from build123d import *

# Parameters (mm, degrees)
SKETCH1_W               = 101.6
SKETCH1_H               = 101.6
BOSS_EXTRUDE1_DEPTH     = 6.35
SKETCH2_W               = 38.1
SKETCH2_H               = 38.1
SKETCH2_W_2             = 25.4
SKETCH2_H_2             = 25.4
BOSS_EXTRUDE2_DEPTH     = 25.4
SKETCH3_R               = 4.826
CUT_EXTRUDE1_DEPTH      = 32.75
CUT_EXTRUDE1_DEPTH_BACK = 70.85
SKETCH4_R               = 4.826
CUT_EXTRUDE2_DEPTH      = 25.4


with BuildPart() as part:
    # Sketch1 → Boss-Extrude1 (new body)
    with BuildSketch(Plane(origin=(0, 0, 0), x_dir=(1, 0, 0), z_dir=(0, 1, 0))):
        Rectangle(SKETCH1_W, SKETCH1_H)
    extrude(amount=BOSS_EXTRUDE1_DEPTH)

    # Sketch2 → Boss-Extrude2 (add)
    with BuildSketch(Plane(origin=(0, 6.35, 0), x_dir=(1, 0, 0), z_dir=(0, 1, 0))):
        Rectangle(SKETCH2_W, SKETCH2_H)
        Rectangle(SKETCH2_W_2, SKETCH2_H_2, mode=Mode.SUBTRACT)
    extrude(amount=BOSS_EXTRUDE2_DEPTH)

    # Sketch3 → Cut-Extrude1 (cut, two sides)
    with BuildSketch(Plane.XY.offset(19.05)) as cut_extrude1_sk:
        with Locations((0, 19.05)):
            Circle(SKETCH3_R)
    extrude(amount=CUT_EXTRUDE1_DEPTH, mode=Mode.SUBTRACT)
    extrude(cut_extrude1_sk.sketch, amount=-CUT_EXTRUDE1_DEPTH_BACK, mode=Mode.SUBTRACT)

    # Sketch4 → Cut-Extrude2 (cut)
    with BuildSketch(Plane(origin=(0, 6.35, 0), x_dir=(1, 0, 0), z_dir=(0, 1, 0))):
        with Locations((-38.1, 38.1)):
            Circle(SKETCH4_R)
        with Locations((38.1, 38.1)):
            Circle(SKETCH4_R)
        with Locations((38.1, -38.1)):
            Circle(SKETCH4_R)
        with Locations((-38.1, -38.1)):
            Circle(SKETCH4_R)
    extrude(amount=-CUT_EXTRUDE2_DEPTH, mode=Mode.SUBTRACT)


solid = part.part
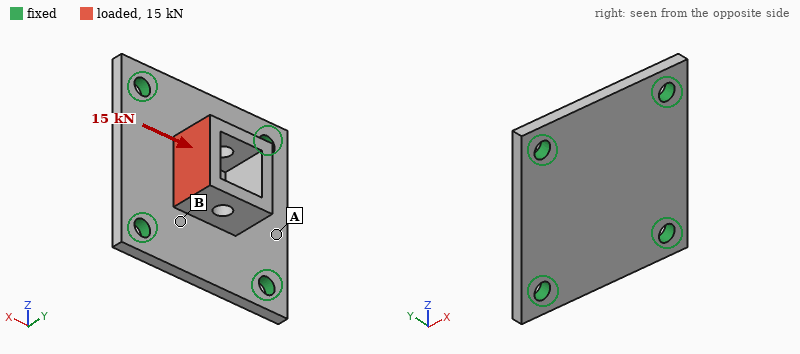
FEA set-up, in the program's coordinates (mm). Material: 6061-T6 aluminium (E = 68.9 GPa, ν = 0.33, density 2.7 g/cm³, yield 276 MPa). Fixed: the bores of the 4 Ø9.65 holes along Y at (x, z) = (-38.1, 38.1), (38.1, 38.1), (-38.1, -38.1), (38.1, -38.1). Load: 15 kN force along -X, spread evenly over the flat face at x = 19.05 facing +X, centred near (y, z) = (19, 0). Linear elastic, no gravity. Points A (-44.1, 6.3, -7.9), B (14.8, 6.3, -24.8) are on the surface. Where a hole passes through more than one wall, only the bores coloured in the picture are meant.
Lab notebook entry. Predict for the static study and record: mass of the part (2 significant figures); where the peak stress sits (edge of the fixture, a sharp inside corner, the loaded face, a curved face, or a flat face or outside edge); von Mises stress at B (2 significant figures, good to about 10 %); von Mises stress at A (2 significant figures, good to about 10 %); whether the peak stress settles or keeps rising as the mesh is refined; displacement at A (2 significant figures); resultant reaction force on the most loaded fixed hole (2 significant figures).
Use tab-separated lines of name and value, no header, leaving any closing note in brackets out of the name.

mass of the part	220 g
where the peak stress sits	edge of the fixture
von Mises stress at B	77 MPa
von Mises stress at A	25 MPa
whether the peak stress settles or keeps rising as the mesh is refined	keeps rising
displacement at A	0.052 mm
resultant reaction force on the most loaded fixed hole	4.6 kN
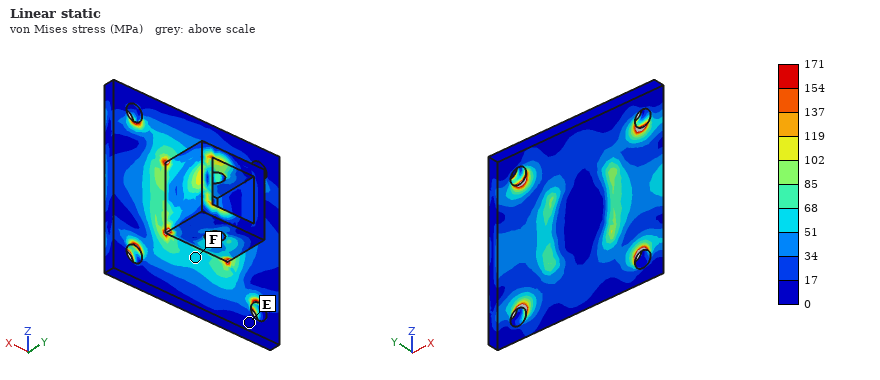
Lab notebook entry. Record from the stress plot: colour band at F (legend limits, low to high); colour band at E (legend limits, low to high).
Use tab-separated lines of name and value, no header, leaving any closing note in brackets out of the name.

colour band at F	51 to 68 MPa
colour band at E	0 to 17 MPa
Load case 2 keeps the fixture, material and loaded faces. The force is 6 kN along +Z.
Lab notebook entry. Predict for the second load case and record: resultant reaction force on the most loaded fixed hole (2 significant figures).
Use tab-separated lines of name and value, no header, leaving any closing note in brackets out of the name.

resultant reaction force on the most loaded fixed hole	2.3 kN
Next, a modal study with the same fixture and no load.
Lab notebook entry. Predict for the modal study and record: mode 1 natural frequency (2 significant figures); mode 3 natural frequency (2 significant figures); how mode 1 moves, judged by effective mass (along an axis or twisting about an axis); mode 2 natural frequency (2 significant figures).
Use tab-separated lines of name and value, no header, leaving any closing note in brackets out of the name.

mode 1 natural frequency	3900 Hz
mode 3 natural frequency	5600 Hz
how mode 1 moves, judged by effective mass	along Y
mode 2 natural frequency	5500 Hz
